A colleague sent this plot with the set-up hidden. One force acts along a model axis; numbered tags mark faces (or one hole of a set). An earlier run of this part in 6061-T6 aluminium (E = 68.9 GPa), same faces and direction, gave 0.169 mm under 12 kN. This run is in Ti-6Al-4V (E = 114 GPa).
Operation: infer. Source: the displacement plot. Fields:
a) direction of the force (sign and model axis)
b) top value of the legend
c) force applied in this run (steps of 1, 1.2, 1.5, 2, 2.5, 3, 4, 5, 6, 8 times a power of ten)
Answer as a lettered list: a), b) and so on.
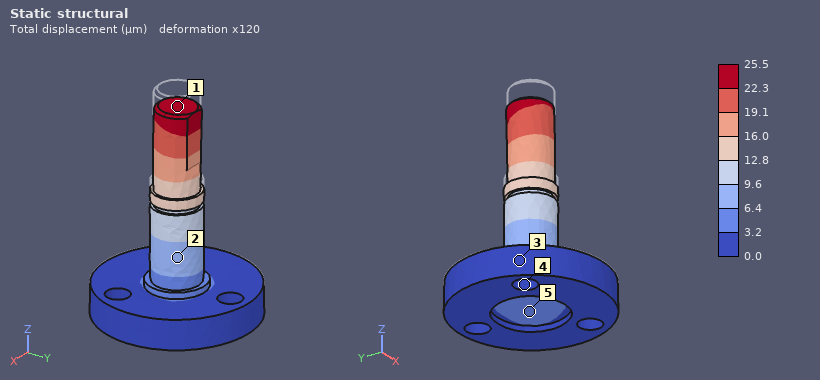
a) -Z
b) 25.5 µm
c) 3 kN
